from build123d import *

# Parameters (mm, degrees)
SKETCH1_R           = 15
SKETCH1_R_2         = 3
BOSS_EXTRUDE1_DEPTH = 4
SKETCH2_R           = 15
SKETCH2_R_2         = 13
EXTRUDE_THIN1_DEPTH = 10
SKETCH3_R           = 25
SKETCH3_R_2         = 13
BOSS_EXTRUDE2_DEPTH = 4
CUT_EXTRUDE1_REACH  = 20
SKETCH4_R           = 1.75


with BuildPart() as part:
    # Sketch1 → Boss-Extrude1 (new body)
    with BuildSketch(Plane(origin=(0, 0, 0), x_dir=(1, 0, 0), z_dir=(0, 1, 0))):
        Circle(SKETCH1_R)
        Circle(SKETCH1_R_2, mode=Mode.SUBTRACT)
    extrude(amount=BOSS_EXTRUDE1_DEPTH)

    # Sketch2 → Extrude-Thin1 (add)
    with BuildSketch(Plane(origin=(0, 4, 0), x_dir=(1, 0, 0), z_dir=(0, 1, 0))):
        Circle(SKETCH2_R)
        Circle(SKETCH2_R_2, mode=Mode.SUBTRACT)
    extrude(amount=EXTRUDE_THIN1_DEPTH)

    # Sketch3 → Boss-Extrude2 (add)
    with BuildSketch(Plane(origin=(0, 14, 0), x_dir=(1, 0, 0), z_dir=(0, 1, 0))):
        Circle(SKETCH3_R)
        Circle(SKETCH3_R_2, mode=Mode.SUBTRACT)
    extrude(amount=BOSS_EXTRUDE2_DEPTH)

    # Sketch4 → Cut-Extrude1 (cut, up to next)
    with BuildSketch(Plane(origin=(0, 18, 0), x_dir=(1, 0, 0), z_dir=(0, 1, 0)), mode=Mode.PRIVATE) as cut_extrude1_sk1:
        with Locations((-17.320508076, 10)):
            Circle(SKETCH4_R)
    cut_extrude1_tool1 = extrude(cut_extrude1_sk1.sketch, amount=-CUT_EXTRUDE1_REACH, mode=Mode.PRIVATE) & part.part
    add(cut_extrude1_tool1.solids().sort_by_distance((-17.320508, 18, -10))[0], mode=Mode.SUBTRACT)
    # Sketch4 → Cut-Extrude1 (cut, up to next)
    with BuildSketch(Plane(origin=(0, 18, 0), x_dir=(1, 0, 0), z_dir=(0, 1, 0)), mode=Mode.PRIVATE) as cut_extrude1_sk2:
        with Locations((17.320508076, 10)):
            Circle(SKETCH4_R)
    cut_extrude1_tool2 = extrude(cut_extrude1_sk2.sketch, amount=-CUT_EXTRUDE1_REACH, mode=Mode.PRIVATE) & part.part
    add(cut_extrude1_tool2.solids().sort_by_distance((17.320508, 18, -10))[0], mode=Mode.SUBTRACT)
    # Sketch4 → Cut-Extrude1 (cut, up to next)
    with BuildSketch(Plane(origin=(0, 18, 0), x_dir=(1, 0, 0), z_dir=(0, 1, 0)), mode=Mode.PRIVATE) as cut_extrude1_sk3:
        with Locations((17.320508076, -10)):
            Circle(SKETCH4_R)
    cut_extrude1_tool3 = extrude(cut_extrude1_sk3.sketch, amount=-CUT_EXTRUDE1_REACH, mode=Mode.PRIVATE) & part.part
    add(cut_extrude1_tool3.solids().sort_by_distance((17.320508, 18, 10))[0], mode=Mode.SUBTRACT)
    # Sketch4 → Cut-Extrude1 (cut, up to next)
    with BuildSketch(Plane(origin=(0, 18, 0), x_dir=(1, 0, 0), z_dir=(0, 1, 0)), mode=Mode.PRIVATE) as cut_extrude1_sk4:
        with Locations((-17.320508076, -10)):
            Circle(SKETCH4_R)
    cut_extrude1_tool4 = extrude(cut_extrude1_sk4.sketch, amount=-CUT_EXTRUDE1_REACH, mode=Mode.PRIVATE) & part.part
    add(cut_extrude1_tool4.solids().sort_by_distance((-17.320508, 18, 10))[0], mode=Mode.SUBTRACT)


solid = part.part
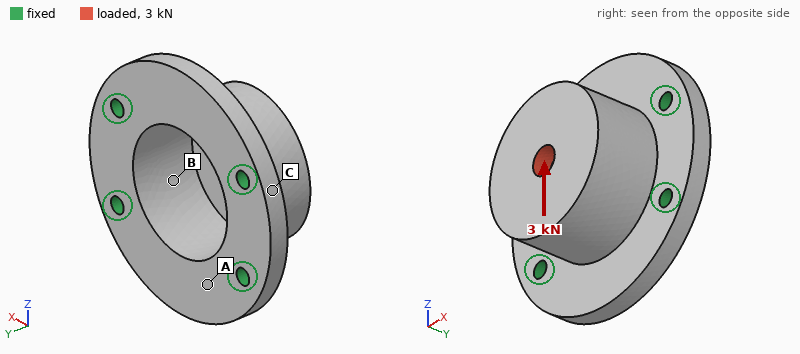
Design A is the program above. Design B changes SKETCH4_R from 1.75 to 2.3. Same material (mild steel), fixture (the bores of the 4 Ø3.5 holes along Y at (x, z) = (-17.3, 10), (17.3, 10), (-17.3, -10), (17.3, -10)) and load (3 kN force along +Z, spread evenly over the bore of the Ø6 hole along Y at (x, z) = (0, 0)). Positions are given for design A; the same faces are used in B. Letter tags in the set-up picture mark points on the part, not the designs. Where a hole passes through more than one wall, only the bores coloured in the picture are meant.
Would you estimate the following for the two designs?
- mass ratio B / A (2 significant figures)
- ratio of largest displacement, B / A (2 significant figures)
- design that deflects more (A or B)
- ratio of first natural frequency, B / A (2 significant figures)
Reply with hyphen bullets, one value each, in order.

- 0.99
- 0.89
- A
- 1.1
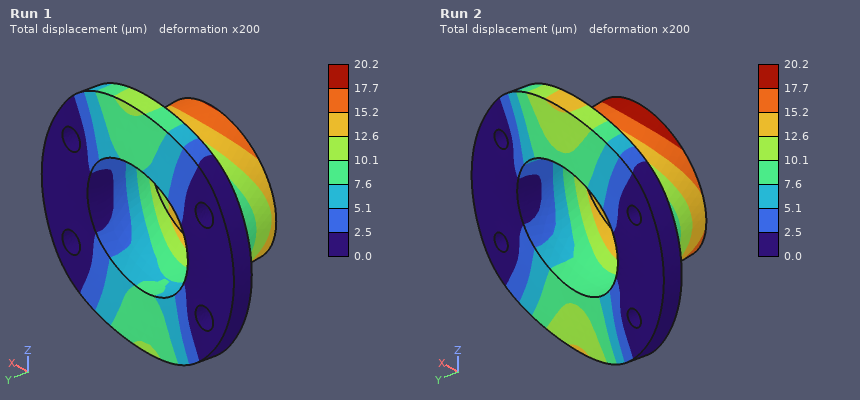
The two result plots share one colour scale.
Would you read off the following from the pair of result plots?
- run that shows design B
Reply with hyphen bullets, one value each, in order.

- Run 1
